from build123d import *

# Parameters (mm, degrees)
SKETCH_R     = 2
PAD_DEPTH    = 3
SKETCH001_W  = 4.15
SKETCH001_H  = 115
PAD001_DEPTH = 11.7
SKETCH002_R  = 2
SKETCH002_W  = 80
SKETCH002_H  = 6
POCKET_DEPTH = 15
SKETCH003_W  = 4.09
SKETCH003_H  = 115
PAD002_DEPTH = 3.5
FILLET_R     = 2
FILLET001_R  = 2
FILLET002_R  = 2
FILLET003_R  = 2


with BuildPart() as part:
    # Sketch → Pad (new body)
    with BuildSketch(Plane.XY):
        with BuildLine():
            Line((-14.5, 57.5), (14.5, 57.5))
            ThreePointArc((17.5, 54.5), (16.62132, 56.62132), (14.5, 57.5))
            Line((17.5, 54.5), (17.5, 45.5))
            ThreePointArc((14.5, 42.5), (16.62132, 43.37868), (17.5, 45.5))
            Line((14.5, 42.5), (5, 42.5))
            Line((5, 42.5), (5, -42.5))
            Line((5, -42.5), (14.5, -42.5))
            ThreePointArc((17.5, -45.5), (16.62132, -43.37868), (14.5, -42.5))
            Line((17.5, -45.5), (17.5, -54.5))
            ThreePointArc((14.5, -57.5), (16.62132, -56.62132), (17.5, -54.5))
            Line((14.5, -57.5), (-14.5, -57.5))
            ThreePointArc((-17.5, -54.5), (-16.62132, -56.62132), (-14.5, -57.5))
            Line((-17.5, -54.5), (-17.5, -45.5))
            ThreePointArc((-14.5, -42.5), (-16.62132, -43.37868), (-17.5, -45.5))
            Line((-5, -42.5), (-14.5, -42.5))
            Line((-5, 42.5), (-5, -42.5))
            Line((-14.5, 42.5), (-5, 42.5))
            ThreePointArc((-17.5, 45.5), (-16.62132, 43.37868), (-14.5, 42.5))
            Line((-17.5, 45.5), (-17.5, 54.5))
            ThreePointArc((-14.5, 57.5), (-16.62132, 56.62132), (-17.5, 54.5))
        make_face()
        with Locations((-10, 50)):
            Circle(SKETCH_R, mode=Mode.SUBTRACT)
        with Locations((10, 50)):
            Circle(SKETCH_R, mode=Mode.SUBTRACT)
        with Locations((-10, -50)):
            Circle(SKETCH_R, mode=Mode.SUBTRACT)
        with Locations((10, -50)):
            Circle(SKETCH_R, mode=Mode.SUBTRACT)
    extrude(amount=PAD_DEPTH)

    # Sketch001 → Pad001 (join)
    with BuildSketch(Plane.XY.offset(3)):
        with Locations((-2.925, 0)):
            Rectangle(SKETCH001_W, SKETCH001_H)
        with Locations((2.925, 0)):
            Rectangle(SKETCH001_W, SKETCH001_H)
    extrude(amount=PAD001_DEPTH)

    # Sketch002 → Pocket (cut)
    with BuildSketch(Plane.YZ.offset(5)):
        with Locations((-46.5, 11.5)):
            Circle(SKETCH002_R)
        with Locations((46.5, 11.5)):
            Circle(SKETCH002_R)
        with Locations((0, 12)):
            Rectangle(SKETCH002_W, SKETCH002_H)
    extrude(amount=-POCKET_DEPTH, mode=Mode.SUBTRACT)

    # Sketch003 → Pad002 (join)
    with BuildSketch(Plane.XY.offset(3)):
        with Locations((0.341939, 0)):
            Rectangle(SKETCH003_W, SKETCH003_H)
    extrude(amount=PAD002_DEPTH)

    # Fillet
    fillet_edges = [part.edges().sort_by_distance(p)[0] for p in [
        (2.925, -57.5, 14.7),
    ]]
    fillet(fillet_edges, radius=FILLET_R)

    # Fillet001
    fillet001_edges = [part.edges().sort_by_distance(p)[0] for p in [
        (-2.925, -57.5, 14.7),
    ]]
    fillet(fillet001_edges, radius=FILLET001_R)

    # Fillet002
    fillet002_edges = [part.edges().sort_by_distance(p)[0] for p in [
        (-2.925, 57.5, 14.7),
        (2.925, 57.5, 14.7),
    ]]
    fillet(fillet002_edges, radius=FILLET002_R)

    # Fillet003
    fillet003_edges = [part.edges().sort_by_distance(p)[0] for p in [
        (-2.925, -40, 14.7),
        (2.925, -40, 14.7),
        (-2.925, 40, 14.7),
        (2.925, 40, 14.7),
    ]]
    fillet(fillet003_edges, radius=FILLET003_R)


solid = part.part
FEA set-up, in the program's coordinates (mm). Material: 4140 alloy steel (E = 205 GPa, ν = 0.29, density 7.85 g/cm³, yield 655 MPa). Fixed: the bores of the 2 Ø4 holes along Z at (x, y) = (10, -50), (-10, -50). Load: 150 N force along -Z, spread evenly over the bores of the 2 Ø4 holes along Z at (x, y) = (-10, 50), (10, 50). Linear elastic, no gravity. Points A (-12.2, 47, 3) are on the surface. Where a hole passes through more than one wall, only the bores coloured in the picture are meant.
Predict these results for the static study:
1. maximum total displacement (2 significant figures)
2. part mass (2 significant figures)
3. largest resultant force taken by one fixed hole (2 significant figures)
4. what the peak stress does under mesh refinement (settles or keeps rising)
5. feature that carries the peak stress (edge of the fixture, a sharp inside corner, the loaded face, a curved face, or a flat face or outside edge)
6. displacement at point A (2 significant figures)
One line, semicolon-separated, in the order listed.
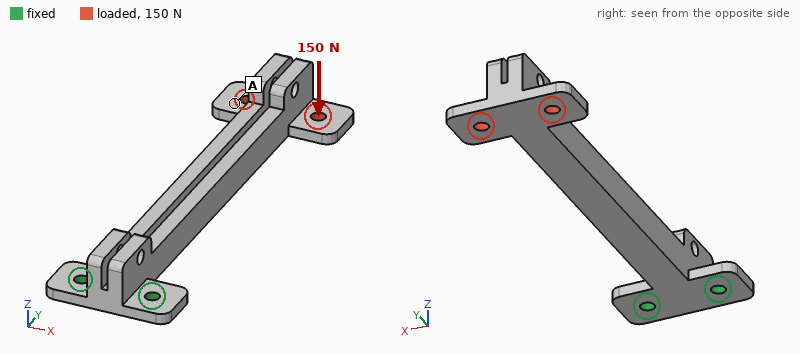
0.72 mm; 100 g; 220 N; keeps rising; edge of the fixture; 0.63 mm
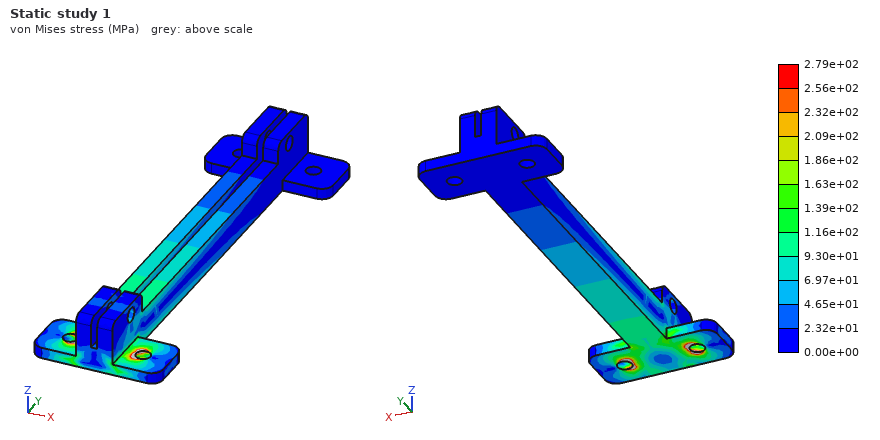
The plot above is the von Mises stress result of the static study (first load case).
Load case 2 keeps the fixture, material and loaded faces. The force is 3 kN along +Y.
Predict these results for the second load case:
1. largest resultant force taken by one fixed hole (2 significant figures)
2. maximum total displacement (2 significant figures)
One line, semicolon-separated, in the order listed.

1.5 kN; 0.38 mm
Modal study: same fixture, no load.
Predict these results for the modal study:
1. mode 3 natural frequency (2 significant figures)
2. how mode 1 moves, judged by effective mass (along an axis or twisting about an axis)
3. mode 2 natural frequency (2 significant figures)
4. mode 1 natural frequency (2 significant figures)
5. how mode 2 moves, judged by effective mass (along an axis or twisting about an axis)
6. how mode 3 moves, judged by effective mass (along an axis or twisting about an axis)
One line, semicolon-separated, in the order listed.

2800 Hz; along Z; 590 Hz; 390 Hz; along X; twisting about Y
